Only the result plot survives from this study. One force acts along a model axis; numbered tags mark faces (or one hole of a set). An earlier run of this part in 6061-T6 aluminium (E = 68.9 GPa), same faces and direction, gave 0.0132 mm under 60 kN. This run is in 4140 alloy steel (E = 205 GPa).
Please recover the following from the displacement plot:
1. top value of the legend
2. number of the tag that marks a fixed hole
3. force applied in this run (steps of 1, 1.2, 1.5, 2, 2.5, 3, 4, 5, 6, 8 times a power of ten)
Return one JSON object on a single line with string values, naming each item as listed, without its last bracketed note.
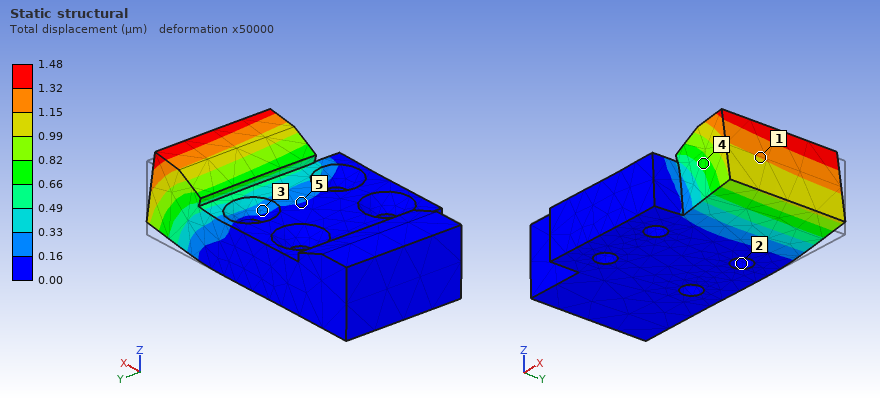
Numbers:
{"top value of the legend": "1.48 µm", "number of the tag that marks a fixed hole": "2", "force applied in this run": "20 kN"}
